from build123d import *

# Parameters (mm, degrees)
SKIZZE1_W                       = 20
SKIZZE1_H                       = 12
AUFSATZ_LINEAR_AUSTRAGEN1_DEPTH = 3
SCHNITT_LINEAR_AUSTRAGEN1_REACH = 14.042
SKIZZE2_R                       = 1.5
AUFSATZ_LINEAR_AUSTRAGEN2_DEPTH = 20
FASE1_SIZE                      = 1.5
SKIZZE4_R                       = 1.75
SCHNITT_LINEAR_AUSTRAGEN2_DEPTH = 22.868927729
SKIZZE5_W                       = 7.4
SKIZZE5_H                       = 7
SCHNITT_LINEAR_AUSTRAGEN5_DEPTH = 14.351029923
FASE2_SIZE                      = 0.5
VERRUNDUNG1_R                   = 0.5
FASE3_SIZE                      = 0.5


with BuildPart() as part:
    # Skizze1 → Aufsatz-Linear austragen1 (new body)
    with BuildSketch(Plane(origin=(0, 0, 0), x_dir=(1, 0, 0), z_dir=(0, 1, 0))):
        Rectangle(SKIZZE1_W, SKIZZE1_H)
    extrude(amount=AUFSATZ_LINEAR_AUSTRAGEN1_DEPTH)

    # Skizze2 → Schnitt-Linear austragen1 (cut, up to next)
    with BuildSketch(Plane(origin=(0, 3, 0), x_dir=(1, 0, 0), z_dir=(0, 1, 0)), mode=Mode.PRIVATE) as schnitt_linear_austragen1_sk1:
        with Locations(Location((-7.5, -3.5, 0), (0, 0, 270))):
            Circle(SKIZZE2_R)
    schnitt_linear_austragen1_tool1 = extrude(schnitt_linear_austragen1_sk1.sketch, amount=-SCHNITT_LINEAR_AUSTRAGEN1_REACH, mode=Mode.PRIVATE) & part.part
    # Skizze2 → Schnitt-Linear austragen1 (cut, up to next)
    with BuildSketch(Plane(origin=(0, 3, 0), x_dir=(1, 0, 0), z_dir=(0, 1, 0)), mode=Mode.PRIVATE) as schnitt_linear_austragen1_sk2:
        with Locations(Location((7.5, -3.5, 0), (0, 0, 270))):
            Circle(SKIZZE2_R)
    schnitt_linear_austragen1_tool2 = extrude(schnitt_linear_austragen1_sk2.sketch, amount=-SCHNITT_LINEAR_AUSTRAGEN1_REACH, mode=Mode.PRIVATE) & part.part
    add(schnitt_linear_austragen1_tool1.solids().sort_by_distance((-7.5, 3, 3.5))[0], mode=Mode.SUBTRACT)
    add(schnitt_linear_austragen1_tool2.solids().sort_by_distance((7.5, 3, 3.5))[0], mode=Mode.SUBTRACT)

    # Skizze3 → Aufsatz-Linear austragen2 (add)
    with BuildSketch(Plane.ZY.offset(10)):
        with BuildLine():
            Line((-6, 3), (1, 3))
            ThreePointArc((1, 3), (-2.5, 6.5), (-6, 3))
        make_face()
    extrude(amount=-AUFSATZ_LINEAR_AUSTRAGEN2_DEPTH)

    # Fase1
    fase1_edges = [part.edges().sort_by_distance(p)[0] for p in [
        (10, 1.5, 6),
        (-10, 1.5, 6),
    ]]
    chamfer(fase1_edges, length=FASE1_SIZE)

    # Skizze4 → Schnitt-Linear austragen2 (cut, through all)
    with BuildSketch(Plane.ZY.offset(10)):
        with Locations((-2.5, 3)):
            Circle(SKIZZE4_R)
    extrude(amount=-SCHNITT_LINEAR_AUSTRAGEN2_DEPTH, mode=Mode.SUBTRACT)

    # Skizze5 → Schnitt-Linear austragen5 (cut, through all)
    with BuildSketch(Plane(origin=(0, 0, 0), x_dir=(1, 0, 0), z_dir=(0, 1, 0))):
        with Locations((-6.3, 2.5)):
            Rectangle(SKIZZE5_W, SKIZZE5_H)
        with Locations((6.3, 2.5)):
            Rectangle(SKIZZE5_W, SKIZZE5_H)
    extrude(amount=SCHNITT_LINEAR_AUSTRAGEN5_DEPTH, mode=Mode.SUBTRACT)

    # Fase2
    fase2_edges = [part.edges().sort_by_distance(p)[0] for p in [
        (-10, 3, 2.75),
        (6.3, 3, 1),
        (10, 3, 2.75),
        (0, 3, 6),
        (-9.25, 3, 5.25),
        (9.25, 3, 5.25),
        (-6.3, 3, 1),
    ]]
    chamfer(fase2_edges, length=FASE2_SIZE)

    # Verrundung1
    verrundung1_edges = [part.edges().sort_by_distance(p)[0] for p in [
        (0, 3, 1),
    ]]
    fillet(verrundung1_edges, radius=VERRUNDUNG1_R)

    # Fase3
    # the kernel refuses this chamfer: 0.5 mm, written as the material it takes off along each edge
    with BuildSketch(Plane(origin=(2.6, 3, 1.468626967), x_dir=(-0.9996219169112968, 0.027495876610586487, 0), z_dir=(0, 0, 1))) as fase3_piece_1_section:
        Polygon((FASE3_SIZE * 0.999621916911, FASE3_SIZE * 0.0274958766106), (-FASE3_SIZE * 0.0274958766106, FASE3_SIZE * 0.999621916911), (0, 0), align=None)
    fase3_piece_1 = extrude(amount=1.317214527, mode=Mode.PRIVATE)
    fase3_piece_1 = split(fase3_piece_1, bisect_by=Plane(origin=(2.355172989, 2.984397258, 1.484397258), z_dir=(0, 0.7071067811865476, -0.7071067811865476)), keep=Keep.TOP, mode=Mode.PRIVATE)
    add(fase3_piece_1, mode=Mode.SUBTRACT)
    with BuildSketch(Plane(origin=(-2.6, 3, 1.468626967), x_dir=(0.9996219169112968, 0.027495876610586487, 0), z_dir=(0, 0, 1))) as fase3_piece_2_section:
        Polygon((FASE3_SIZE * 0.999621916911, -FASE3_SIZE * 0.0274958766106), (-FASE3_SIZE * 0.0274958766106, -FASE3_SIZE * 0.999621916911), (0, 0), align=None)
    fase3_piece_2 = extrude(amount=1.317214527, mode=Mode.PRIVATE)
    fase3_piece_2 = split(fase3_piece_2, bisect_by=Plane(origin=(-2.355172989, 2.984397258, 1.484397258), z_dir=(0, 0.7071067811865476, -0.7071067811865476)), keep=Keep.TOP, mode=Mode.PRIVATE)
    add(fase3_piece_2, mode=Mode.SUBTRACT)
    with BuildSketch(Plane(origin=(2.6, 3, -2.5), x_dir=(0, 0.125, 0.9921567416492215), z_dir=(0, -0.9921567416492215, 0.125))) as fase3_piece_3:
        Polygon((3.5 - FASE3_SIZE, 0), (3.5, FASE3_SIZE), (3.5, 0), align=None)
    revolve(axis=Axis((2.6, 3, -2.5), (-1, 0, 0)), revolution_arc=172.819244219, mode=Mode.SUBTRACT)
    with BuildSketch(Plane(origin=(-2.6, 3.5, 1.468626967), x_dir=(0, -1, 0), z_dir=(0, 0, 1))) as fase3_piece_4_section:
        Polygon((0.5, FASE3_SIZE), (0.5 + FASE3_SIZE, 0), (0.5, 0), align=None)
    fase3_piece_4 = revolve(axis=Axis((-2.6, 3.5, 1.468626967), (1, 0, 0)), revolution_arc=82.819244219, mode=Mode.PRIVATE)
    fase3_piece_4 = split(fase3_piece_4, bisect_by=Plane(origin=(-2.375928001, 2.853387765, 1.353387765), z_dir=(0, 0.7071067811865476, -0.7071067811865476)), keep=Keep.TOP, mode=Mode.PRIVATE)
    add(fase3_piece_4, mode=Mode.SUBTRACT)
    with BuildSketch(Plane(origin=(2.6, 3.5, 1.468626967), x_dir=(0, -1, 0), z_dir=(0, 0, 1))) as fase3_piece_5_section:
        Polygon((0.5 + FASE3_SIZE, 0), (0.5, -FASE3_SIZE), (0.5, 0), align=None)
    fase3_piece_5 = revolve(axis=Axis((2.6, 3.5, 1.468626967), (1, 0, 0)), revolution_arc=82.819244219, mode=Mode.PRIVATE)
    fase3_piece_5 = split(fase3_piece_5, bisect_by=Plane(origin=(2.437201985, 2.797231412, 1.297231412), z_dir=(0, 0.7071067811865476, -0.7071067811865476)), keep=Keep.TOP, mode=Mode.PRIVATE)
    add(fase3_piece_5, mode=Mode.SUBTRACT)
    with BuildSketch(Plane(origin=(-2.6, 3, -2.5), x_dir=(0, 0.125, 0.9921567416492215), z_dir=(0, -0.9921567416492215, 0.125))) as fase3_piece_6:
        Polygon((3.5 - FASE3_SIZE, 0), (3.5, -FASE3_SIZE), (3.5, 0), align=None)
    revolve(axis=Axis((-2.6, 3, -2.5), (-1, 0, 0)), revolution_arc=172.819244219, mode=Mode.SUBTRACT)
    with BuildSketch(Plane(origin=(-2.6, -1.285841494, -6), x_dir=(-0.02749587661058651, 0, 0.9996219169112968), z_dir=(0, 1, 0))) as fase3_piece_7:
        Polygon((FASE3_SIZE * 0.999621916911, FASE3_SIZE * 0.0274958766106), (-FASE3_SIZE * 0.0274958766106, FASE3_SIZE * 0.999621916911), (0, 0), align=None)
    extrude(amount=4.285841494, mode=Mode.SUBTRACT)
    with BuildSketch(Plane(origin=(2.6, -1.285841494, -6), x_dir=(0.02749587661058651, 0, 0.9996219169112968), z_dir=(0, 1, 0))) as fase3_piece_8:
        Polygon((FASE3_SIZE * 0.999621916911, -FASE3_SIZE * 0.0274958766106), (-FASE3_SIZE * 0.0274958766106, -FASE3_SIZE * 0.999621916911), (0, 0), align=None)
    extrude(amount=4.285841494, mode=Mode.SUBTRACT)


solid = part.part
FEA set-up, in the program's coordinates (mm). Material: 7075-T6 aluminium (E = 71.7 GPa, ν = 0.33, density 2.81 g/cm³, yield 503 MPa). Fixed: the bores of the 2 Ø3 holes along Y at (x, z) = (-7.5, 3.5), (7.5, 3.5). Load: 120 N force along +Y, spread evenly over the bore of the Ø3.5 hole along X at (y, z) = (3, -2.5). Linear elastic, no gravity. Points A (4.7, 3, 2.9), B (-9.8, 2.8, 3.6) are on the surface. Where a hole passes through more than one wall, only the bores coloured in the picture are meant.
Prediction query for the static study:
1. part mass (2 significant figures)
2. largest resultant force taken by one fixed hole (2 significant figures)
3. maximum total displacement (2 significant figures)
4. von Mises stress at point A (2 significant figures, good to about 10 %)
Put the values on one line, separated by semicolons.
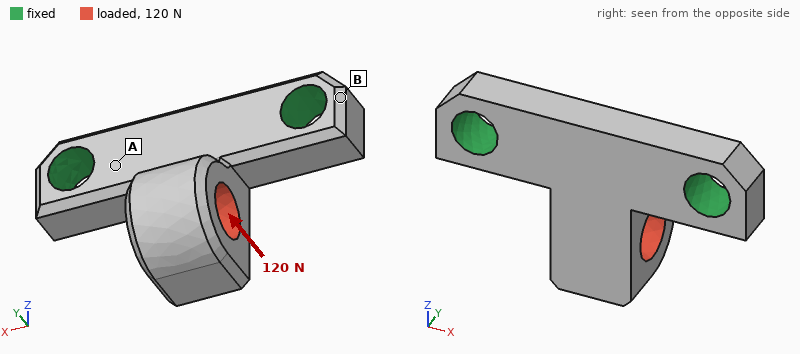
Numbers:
1.1 g; 60 N; 38 µm; 53 MPa
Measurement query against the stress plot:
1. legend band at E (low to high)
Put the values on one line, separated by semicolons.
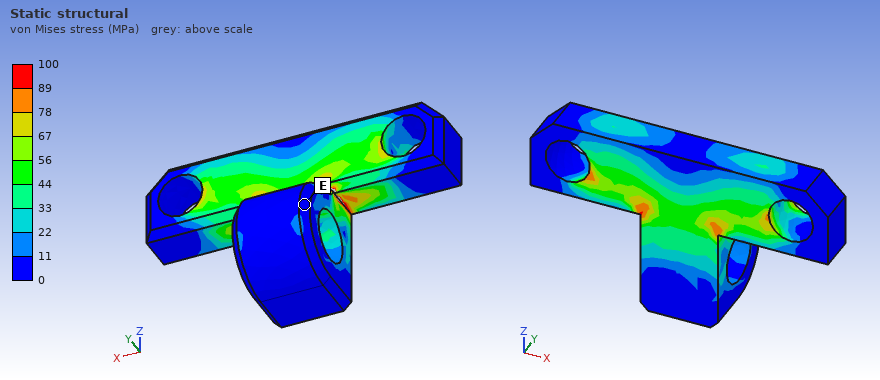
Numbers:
0 to 11 MPa
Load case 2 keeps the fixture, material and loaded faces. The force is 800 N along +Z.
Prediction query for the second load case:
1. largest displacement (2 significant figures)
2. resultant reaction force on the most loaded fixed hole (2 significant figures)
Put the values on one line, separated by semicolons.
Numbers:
78 µm; 410 N
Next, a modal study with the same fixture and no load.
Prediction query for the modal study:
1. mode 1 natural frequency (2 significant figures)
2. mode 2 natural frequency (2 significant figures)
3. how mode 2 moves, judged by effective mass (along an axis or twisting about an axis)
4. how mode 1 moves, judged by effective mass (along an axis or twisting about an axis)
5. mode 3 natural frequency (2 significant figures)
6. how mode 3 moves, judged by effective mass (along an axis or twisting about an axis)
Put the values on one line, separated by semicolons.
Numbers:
15 kHz; 33 kHz; along X; along Y; 51 kHz; along Z
